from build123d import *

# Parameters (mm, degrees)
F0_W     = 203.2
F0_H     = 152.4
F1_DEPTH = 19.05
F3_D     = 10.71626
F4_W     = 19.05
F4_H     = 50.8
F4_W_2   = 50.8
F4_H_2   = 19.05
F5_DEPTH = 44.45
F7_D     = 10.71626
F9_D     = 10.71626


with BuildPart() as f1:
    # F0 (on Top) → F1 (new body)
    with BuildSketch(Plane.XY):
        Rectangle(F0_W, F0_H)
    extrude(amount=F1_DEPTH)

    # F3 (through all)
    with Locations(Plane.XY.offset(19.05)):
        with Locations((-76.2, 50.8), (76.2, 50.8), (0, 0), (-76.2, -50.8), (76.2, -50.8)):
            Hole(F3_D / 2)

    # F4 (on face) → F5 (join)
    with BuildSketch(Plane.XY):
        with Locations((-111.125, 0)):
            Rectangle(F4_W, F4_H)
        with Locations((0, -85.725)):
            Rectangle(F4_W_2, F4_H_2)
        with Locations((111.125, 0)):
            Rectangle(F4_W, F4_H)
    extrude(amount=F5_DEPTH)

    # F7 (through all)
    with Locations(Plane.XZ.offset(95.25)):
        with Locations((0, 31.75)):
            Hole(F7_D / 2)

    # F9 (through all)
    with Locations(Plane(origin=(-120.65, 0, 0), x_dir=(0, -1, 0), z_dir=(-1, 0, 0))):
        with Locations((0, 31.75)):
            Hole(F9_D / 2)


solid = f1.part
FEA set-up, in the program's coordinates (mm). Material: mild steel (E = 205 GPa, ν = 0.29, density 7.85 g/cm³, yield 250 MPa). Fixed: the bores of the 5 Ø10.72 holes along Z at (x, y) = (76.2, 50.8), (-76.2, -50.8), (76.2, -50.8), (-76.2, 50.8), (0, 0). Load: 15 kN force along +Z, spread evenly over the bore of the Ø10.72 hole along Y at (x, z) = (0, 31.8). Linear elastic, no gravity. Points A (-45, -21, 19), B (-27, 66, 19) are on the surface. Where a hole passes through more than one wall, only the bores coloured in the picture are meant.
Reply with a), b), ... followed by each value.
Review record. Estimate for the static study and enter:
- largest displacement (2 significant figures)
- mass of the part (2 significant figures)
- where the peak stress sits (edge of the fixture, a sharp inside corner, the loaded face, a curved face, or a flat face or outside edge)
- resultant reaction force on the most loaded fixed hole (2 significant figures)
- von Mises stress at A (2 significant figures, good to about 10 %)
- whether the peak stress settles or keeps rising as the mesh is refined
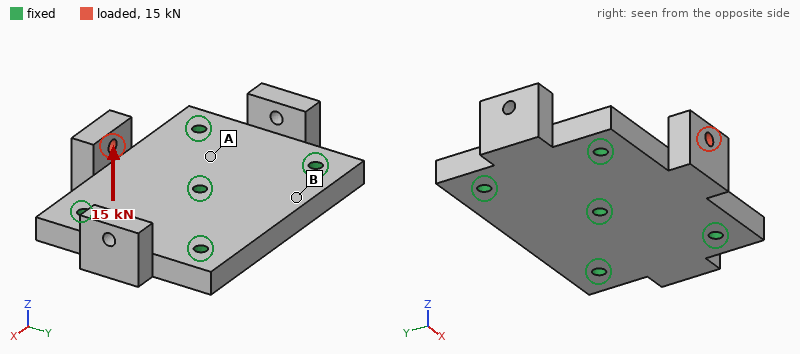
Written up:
a) 0.15 mm
b) 5.5 kg
c) edge of the fixture
d) 7.6 kN
e) 32 MPa
f) keeps rising
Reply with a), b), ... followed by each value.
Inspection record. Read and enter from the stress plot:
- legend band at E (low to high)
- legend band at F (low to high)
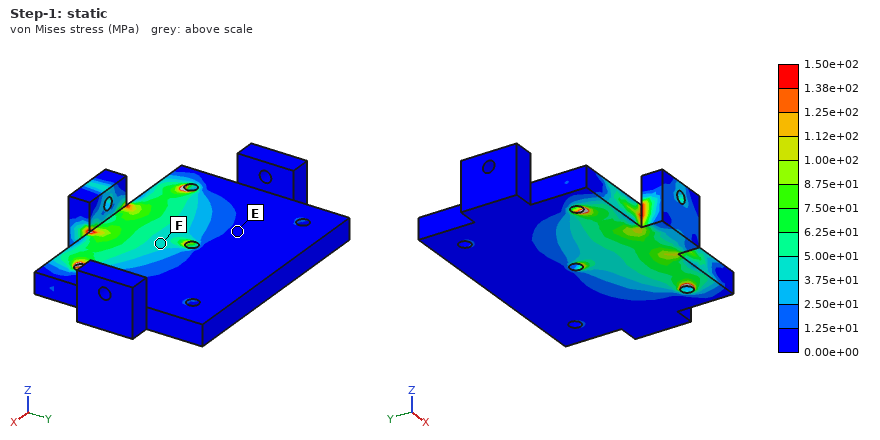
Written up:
a) 0.00e+00 to 1.25e+01 MPa
b) 3.75e+01 to 5.00e+01 MPa
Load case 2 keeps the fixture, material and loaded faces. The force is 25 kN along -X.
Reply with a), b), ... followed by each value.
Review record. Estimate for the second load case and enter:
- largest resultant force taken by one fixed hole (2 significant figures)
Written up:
a) 13 kN
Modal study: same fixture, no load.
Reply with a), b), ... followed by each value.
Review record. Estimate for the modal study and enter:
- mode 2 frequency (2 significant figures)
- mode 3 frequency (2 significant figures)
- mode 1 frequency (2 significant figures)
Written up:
a) 3700 Hz
b) 3700 Hz
c) 2800 Hz
